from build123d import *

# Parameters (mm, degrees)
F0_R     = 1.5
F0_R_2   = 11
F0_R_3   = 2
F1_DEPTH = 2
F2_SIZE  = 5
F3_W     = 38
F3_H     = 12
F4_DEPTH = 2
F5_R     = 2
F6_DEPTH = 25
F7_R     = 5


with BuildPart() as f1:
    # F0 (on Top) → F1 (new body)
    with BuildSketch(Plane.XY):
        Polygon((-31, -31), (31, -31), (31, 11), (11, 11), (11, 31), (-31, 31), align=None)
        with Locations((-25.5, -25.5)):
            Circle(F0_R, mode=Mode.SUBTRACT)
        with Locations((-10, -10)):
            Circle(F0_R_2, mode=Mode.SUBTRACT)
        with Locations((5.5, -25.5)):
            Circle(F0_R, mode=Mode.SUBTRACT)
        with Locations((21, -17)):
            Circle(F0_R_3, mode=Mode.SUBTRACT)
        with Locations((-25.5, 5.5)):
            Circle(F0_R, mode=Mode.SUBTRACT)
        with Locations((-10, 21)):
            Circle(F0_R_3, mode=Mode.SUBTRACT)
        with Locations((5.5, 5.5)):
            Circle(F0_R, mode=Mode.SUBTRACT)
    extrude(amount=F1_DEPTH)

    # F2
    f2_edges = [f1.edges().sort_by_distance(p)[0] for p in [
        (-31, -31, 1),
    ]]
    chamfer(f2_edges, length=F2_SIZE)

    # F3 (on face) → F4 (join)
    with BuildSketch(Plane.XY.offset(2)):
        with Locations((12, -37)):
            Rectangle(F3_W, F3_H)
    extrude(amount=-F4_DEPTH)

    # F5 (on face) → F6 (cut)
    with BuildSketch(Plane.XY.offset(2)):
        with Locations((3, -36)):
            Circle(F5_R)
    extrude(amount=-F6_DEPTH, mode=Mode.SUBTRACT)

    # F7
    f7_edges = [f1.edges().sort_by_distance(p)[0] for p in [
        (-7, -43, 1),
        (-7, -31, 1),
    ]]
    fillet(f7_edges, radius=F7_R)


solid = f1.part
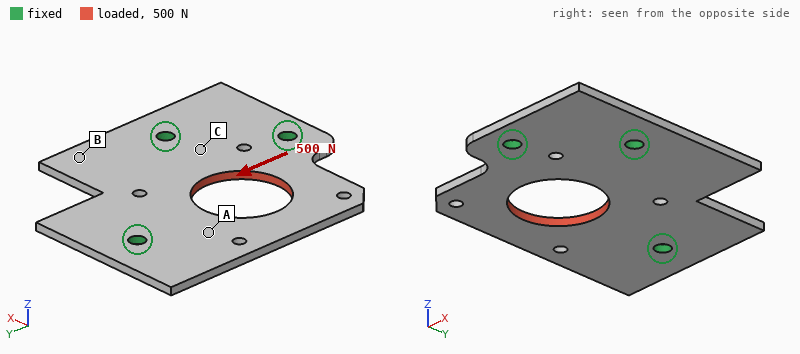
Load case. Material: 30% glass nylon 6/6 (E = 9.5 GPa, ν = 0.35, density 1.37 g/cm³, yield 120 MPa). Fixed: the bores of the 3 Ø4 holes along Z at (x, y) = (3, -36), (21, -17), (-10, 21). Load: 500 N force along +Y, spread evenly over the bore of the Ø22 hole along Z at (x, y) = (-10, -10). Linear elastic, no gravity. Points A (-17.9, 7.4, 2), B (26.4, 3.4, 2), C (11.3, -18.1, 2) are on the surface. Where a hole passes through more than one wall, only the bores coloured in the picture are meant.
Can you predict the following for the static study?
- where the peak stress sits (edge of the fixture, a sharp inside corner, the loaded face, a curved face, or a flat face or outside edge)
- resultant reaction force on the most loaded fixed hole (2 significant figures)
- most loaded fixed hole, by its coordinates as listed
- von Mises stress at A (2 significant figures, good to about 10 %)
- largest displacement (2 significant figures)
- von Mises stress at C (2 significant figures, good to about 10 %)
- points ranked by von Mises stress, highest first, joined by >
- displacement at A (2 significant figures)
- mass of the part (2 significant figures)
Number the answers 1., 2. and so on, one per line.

1. edge of the fixture
2. 260 N
3. (-10, 21)
4. 7.1 MPa
5. 35 µm
6. 3.1 MPa
7. A > C > B
8. 17 µm
9. 9.4 g
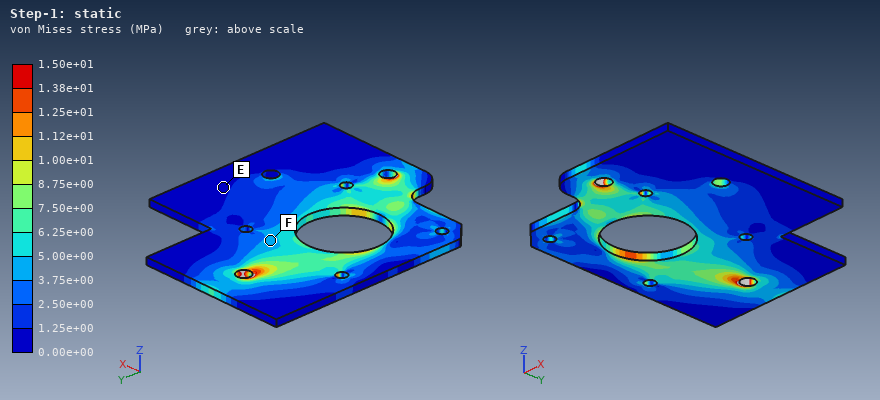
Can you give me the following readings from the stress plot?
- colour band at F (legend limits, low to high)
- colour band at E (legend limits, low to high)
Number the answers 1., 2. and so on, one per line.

1. 3.75e+00 to 5.00e+00 MPa
2. 0.00e+00 to 1.25e+00 MPa
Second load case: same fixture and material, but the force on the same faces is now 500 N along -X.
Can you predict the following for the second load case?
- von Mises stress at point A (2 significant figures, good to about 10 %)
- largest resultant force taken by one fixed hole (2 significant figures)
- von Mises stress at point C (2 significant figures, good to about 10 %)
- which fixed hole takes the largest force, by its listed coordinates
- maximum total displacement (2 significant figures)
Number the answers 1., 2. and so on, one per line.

1. 3.9 MPa
2. 210 N
3. 6.7 MPa
4. (21, -17)
5. 38 µm
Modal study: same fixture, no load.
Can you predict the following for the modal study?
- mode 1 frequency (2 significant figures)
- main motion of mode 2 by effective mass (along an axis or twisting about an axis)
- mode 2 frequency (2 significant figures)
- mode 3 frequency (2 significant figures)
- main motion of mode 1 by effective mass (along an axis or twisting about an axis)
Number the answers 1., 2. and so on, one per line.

1. 880 Hz
2. along Z
3. 1600 Hz
4. 2000 Hz
5. along Z
